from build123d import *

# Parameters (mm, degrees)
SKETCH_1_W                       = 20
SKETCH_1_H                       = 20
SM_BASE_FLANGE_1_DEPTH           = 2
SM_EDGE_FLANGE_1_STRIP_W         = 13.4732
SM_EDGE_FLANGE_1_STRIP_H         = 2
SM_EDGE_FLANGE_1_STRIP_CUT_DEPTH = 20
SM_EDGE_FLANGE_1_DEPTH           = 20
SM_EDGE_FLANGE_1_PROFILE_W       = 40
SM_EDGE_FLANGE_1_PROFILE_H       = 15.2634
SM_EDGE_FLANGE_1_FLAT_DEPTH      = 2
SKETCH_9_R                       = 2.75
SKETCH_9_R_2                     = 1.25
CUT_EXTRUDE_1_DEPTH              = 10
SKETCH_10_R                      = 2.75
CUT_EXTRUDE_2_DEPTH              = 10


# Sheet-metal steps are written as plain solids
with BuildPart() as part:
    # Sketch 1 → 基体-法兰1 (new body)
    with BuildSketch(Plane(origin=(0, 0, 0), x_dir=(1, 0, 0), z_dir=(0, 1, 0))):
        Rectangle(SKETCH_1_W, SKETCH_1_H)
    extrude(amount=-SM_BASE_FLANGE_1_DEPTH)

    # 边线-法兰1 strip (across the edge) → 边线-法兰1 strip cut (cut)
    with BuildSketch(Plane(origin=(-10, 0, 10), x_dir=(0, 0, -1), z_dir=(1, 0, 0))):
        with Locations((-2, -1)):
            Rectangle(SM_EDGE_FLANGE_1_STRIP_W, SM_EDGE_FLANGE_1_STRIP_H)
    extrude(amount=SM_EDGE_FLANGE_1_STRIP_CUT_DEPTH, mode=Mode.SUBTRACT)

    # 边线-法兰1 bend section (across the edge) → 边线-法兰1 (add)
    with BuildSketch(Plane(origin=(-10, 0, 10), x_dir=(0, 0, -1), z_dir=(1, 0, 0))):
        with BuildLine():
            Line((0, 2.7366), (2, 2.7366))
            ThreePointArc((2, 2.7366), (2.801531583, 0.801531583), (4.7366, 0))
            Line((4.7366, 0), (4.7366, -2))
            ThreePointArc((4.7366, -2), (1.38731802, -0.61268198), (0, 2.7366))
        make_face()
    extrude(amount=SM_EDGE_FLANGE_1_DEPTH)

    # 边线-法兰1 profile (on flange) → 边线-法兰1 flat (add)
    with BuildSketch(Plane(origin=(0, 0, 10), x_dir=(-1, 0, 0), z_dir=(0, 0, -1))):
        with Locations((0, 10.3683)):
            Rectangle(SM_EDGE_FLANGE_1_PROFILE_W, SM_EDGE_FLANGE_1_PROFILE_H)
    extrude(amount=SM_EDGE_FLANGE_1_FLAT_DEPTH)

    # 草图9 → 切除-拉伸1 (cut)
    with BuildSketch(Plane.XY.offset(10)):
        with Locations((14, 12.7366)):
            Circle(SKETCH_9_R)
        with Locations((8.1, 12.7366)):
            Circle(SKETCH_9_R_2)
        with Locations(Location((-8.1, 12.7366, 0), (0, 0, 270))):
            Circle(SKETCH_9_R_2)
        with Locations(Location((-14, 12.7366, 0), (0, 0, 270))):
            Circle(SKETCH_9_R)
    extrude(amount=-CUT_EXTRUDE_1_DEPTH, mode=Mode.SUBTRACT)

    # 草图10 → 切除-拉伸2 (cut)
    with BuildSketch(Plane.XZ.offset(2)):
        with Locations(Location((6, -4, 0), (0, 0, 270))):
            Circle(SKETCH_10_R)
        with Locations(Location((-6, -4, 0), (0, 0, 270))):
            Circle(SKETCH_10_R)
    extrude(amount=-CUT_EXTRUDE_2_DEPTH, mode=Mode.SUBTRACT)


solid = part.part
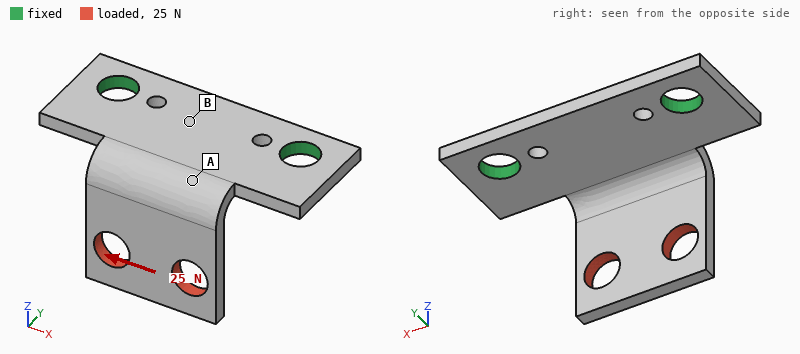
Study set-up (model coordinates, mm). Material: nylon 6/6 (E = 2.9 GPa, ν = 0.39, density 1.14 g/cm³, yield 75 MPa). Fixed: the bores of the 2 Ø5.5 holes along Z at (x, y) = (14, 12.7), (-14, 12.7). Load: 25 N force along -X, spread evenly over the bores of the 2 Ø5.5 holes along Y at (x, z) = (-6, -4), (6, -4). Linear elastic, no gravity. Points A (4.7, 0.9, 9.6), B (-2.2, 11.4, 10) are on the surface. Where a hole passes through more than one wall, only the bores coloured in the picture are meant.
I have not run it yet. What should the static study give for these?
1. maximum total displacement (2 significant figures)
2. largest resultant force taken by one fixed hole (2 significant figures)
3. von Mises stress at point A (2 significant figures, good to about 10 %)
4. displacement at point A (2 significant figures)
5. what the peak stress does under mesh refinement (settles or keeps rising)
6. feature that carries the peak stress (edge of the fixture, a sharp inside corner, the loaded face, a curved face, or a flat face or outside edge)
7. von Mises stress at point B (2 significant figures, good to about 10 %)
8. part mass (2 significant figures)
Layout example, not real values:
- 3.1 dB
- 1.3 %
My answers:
- 0.50 mm
- 22 N
- 7.4 MPa
- 0.083 mm
- keeps rising
- a sharp inside corner
- 2.4 MPa
- 2.1 g
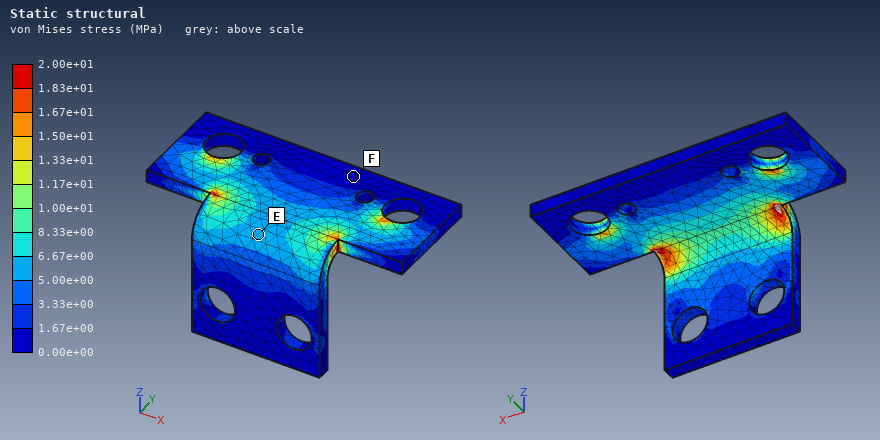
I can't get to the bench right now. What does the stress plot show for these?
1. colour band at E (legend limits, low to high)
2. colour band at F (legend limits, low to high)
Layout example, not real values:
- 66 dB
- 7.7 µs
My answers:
- 5.00e+00 to 6.67e+00 MPa
- 0.00e+00 to 1.67e+00 MPa
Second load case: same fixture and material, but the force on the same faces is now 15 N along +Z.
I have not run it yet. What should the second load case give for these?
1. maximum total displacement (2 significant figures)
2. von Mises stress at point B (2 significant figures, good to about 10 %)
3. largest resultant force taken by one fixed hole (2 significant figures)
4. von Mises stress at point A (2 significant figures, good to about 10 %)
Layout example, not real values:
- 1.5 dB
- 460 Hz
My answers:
- 0.50 mm
- 2.6 MPa
- 7.5 N
- 2.6 MPa
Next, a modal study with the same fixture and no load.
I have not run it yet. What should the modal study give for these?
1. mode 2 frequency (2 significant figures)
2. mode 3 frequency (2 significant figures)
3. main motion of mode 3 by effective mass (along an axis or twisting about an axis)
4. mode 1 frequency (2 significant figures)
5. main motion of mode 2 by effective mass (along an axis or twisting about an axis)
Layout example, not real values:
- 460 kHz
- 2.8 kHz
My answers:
- 1800 Hz
- 2200 Hz
- along Z
- 850 Hz
- along X
